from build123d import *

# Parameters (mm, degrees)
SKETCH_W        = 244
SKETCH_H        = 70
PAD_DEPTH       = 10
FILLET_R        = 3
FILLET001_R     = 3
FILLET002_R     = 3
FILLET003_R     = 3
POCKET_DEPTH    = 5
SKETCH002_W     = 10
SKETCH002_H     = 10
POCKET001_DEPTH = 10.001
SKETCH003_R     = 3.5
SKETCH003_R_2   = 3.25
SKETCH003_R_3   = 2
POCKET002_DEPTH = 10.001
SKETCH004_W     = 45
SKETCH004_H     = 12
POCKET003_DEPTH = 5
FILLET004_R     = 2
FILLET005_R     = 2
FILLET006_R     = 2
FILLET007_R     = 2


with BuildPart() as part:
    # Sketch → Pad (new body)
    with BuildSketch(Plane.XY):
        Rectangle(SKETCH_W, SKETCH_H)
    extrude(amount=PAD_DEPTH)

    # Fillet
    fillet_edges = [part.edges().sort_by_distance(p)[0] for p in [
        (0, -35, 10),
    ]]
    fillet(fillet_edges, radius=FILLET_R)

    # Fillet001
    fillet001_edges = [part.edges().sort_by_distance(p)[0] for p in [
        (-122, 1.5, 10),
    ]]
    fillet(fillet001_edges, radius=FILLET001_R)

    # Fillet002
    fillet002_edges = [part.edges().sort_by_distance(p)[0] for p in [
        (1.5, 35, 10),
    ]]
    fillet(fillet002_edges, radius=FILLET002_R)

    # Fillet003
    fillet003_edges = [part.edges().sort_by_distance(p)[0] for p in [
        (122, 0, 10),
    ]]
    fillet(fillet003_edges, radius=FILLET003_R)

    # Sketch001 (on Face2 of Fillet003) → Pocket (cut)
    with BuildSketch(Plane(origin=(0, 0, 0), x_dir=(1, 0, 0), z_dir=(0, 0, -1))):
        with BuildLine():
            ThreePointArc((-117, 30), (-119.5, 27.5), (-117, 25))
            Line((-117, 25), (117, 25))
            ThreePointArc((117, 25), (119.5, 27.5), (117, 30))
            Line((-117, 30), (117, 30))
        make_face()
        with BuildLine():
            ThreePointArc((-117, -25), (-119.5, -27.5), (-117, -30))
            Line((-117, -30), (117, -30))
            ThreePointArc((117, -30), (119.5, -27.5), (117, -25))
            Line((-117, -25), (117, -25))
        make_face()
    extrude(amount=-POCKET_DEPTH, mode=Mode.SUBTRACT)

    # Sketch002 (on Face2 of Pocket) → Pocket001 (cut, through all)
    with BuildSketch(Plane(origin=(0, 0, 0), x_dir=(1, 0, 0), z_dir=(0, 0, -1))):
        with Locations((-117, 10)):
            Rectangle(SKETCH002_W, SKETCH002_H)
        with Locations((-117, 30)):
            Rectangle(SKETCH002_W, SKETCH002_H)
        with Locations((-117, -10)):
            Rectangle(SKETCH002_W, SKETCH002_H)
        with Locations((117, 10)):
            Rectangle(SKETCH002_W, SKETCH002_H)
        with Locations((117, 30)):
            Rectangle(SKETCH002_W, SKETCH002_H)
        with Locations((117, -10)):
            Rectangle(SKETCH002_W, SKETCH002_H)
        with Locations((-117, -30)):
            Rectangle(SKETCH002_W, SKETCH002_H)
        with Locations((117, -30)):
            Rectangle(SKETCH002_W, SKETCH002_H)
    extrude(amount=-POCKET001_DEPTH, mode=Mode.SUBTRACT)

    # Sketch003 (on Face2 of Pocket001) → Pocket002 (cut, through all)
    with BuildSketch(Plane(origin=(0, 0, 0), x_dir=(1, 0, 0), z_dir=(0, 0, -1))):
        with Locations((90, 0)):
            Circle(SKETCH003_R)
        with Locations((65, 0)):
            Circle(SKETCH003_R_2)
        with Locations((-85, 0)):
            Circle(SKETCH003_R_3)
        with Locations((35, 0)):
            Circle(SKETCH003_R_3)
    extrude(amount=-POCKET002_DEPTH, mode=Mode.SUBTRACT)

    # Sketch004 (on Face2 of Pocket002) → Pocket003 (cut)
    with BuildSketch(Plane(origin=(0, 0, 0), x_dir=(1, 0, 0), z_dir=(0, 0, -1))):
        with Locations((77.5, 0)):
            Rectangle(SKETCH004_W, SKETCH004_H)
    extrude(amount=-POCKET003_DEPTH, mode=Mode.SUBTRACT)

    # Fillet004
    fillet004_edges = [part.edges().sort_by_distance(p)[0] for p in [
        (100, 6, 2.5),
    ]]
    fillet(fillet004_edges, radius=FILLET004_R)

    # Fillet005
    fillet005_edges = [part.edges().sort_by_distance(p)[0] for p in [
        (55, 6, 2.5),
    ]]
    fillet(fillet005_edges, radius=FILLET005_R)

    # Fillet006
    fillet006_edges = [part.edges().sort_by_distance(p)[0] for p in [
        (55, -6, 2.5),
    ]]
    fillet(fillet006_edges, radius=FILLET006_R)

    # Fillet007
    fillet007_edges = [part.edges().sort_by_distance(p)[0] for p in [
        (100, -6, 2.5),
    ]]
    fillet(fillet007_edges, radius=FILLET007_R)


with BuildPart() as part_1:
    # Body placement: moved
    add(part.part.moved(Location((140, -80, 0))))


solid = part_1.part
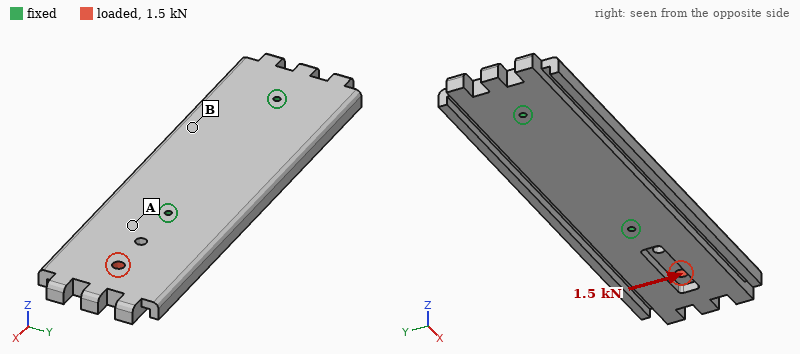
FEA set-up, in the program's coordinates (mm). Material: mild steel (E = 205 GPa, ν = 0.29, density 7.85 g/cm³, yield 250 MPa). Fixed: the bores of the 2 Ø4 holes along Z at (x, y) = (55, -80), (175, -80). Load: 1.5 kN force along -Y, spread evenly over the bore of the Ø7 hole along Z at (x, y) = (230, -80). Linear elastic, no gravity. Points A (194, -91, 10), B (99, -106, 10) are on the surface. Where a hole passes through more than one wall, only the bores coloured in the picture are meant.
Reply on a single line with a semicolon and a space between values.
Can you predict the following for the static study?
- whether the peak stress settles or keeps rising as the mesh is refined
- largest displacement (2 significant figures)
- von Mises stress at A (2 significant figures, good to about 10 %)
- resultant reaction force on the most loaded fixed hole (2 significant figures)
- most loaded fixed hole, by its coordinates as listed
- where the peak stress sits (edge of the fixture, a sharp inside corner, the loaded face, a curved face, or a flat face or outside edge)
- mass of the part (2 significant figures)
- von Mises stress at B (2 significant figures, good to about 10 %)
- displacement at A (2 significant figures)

keeps rising; 15 µm; 6.9 MPa; 2.2 kN; (175, -80); edge of the fixture; 1.2 kg; 3.4 MPa; 3.5 µm
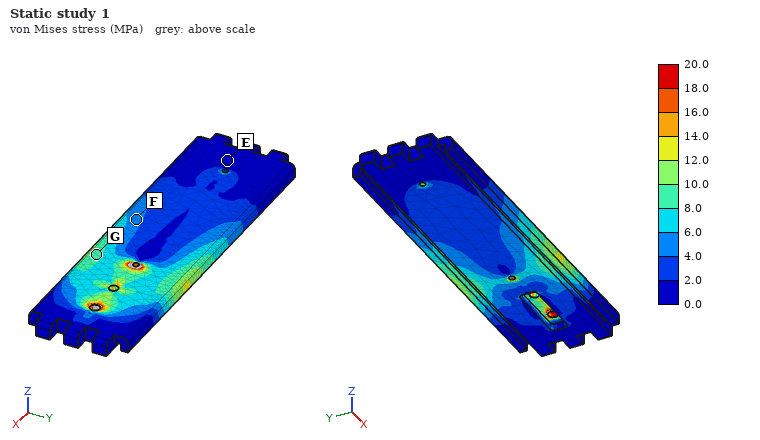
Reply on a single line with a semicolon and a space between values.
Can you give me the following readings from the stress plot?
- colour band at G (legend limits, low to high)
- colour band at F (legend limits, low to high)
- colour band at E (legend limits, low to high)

8.0 to 10.0 MPa; 4.0 to 6.0 MPa; 0.0 to 2.0 MPa
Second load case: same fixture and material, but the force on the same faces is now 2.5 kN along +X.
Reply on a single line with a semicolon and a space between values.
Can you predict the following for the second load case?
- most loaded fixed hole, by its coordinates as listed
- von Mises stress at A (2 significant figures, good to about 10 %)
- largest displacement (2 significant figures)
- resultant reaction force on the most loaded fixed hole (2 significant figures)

(175, -80); 11 MPa; 22 µm; 2.0 kN
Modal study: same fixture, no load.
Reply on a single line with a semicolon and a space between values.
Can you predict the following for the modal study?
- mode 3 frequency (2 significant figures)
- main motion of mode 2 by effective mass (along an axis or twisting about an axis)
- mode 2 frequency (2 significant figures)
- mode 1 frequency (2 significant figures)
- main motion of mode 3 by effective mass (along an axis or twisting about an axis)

2600 Hz; twisting about X; 2000 Hz; 1000 Hz; along Z
